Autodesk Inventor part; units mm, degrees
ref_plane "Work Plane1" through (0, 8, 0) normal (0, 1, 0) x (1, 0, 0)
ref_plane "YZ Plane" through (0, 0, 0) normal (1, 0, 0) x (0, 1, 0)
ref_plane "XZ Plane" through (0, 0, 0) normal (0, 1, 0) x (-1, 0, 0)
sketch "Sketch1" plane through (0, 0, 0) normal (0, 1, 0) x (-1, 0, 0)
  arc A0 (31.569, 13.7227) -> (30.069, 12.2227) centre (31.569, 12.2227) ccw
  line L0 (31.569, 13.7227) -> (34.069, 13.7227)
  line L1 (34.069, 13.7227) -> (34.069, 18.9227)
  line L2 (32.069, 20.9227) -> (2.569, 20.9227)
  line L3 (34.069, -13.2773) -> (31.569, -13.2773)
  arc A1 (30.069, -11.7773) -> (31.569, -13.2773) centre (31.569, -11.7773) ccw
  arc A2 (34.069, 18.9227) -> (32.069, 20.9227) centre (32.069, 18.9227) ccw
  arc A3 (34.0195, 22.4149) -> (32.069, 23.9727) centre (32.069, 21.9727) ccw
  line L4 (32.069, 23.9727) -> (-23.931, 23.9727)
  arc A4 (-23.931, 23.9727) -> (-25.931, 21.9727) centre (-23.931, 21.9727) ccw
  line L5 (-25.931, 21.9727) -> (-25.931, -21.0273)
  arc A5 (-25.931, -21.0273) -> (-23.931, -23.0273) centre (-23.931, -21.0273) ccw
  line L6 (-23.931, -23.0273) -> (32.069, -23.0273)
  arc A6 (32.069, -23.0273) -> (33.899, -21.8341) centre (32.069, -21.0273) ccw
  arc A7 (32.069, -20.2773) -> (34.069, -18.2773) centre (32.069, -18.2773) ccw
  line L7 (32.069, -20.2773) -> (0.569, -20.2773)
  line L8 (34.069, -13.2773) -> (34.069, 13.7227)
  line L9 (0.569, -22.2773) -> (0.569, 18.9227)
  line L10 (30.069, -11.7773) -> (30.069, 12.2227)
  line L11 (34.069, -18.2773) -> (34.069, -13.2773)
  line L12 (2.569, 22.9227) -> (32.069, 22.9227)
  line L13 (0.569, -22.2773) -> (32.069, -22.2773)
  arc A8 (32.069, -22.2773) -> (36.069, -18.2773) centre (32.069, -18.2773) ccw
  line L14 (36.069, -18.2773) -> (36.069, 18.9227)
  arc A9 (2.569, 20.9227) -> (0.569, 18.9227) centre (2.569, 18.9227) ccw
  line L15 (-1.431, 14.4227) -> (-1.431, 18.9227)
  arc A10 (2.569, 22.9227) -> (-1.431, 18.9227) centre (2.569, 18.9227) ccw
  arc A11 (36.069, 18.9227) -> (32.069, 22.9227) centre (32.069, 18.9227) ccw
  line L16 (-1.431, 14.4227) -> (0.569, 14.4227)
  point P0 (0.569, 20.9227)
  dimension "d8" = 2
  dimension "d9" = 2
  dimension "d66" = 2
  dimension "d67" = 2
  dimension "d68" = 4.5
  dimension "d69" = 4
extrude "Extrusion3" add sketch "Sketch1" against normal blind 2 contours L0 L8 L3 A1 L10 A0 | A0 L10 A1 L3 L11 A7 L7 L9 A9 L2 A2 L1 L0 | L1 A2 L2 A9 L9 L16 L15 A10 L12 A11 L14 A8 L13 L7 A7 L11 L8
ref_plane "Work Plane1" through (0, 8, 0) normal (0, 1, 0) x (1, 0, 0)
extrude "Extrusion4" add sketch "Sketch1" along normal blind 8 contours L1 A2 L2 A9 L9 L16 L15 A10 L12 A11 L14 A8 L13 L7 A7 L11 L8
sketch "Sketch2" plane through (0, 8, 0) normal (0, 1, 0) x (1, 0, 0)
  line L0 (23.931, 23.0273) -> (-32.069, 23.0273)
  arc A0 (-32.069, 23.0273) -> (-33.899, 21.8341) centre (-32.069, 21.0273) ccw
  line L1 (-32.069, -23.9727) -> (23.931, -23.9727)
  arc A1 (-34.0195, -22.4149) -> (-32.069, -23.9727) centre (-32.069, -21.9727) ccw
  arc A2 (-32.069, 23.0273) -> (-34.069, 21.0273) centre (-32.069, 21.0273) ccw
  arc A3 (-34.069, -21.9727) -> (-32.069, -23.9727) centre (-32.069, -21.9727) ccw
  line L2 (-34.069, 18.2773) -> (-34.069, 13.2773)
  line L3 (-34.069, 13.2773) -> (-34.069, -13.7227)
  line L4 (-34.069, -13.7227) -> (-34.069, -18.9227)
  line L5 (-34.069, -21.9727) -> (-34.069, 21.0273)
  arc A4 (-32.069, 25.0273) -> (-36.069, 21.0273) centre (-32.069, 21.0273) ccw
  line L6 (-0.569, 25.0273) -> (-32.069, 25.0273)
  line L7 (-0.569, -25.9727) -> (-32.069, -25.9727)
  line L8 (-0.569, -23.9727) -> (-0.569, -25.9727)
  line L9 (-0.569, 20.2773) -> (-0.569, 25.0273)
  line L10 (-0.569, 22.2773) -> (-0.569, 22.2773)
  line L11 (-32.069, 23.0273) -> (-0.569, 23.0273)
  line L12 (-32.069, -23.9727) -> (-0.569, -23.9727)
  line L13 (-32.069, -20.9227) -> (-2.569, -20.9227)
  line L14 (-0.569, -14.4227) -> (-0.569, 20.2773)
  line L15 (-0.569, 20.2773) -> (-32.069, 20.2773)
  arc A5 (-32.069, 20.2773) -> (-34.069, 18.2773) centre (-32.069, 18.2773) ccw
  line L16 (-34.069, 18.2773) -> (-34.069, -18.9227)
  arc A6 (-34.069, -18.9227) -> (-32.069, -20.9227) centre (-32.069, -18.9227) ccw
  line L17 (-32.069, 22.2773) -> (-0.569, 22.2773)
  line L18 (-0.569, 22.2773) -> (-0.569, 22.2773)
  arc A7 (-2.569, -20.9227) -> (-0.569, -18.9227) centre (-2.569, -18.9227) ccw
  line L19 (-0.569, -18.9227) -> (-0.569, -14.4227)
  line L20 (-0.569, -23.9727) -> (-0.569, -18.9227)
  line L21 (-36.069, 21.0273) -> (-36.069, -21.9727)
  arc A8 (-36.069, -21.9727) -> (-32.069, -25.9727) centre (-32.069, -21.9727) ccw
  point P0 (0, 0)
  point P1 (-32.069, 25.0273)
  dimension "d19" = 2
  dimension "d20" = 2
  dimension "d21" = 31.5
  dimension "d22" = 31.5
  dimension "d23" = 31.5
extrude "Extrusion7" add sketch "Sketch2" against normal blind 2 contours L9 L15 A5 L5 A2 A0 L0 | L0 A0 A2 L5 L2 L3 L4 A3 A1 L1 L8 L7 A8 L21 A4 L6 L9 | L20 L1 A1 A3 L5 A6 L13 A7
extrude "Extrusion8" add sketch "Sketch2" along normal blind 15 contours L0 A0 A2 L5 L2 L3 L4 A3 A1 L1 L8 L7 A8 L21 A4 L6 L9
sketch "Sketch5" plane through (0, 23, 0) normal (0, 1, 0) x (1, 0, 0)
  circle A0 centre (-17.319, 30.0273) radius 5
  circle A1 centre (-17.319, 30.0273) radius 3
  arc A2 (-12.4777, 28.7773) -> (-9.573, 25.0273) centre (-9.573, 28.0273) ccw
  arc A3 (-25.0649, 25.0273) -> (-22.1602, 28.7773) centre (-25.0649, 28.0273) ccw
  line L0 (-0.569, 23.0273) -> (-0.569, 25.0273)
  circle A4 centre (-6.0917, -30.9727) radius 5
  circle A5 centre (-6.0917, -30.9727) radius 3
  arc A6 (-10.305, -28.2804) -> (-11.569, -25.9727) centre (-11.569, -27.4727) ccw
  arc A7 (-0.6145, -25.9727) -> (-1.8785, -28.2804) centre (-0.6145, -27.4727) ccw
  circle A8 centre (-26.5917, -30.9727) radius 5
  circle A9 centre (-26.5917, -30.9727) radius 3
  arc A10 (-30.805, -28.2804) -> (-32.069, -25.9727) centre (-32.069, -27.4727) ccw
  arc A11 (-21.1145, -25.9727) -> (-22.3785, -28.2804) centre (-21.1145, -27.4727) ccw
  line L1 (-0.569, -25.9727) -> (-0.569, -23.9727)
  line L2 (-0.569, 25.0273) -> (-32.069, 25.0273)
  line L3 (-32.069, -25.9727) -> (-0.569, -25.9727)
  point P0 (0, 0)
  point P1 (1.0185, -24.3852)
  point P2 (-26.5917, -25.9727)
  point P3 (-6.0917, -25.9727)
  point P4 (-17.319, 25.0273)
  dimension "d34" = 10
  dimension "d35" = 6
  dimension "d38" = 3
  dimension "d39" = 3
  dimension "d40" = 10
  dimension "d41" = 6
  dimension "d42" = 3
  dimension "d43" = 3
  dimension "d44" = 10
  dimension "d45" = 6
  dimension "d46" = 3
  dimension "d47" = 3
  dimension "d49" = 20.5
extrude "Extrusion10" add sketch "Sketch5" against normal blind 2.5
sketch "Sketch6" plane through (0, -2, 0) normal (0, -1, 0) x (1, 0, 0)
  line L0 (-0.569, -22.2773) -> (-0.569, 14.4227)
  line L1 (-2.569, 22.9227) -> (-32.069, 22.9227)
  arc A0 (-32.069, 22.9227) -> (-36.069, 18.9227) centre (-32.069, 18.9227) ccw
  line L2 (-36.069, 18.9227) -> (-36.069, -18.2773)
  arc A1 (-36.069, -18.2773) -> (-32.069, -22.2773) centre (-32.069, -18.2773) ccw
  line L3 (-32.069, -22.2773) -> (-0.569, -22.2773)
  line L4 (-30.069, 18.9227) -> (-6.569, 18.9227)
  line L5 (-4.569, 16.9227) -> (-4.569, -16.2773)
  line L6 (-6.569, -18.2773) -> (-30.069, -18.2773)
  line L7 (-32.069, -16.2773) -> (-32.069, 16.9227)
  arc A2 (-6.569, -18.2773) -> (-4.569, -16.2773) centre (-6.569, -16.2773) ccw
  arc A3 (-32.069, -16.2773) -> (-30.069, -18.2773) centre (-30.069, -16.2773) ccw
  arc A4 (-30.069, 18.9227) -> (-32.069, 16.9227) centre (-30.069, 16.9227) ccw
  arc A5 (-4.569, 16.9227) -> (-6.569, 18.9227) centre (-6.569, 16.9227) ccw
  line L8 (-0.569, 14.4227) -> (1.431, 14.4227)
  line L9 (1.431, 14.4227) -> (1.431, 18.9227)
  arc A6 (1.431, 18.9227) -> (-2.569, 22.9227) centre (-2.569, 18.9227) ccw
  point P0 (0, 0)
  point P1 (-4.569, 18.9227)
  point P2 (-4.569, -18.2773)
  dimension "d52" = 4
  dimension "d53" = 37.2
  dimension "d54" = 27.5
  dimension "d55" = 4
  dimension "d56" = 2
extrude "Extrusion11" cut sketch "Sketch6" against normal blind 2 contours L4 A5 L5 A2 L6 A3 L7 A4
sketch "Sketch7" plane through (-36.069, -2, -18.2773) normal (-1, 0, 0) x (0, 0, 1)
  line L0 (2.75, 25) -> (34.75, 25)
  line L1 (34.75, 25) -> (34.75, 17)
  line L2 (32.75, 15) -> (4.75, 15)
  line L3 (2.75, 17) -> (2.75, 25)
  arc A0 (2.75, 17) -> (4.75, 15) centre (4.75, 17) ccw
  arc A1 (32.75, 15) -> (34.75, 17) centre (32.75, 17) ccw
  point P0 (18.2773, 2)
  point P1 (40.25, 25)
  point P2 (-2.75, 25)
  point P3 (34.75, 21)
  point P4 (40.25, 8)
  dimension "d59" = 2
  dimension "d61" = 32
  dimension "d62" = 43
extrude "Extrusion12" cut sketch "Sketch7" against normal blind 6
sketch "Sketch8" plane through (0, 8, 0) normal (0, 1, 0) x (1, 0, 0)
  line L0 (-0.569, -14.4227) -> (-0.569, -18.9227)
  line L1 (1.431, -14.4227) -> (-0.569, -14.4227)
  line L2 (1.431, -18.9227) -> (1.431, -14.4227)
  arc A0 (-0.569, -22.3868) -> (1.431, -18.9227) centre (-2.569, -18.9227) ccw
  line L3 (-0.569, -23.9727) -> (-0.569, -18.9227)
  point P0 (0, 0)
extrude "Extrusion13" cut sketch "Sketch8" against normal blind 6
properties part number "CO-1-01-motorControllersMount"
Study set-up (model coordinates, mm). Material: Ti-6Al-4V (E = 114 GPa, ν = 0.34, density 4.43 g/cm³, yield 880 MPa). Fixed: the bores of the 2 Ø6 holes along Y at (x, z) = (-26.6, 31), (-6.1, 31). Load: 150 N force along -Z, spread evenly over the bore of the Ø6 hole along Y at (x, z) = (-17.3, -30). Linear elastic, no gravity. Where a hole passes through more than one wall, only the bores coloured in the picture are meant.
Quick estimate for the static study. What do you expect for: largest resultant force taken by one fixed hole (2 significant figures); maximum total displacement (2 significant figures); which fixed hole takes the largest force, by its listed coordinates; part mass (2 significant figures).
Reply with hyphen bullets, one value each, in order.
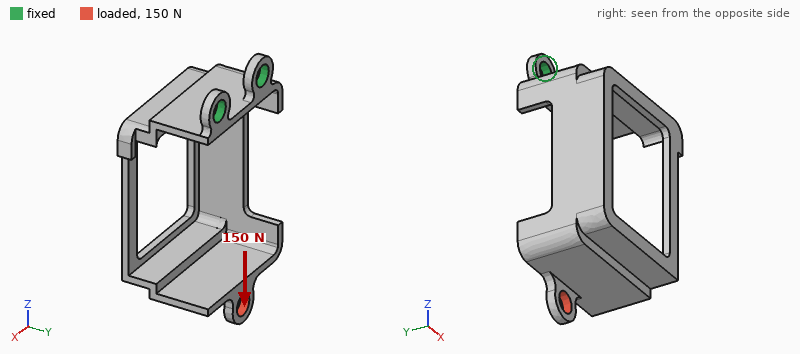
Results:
- 92 N
- 0.83 mm
- (-6.1, 31)
- 29 g
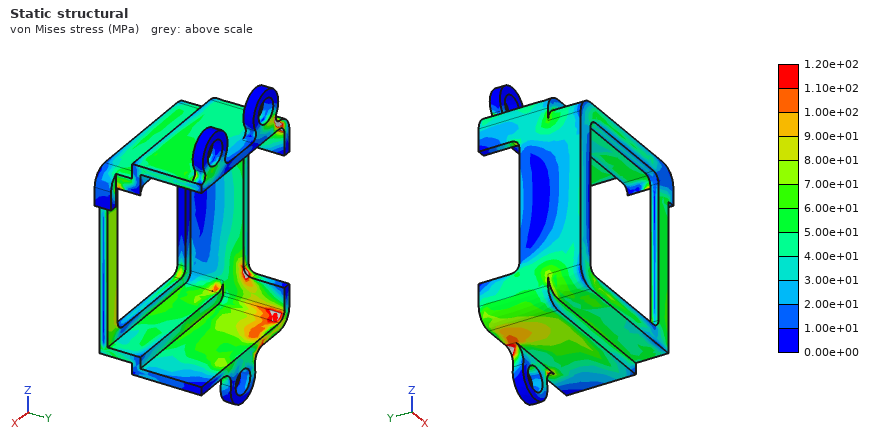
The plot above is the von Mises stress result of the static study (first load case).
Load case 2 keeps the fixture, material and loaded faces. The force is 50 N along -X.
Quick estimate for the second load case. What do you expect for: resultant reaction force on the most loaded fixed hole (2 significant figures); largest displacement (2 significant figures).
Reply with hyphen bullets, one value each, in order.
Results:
- 100 N
- 0.85 mm
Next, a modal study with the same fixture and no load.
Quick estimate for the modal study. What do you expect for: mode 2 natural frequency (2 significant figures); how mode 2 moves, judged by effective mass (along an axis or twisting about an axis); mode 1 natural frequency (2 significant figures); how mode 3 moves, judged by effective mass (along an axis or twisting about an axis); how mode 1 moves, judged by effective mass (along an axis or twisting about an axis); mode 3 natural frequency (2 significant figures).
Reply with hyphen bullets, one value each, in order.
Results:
- 470 Hz
- along X
- 360 Hz
- along Z
- along Y
- 1200 Hz
